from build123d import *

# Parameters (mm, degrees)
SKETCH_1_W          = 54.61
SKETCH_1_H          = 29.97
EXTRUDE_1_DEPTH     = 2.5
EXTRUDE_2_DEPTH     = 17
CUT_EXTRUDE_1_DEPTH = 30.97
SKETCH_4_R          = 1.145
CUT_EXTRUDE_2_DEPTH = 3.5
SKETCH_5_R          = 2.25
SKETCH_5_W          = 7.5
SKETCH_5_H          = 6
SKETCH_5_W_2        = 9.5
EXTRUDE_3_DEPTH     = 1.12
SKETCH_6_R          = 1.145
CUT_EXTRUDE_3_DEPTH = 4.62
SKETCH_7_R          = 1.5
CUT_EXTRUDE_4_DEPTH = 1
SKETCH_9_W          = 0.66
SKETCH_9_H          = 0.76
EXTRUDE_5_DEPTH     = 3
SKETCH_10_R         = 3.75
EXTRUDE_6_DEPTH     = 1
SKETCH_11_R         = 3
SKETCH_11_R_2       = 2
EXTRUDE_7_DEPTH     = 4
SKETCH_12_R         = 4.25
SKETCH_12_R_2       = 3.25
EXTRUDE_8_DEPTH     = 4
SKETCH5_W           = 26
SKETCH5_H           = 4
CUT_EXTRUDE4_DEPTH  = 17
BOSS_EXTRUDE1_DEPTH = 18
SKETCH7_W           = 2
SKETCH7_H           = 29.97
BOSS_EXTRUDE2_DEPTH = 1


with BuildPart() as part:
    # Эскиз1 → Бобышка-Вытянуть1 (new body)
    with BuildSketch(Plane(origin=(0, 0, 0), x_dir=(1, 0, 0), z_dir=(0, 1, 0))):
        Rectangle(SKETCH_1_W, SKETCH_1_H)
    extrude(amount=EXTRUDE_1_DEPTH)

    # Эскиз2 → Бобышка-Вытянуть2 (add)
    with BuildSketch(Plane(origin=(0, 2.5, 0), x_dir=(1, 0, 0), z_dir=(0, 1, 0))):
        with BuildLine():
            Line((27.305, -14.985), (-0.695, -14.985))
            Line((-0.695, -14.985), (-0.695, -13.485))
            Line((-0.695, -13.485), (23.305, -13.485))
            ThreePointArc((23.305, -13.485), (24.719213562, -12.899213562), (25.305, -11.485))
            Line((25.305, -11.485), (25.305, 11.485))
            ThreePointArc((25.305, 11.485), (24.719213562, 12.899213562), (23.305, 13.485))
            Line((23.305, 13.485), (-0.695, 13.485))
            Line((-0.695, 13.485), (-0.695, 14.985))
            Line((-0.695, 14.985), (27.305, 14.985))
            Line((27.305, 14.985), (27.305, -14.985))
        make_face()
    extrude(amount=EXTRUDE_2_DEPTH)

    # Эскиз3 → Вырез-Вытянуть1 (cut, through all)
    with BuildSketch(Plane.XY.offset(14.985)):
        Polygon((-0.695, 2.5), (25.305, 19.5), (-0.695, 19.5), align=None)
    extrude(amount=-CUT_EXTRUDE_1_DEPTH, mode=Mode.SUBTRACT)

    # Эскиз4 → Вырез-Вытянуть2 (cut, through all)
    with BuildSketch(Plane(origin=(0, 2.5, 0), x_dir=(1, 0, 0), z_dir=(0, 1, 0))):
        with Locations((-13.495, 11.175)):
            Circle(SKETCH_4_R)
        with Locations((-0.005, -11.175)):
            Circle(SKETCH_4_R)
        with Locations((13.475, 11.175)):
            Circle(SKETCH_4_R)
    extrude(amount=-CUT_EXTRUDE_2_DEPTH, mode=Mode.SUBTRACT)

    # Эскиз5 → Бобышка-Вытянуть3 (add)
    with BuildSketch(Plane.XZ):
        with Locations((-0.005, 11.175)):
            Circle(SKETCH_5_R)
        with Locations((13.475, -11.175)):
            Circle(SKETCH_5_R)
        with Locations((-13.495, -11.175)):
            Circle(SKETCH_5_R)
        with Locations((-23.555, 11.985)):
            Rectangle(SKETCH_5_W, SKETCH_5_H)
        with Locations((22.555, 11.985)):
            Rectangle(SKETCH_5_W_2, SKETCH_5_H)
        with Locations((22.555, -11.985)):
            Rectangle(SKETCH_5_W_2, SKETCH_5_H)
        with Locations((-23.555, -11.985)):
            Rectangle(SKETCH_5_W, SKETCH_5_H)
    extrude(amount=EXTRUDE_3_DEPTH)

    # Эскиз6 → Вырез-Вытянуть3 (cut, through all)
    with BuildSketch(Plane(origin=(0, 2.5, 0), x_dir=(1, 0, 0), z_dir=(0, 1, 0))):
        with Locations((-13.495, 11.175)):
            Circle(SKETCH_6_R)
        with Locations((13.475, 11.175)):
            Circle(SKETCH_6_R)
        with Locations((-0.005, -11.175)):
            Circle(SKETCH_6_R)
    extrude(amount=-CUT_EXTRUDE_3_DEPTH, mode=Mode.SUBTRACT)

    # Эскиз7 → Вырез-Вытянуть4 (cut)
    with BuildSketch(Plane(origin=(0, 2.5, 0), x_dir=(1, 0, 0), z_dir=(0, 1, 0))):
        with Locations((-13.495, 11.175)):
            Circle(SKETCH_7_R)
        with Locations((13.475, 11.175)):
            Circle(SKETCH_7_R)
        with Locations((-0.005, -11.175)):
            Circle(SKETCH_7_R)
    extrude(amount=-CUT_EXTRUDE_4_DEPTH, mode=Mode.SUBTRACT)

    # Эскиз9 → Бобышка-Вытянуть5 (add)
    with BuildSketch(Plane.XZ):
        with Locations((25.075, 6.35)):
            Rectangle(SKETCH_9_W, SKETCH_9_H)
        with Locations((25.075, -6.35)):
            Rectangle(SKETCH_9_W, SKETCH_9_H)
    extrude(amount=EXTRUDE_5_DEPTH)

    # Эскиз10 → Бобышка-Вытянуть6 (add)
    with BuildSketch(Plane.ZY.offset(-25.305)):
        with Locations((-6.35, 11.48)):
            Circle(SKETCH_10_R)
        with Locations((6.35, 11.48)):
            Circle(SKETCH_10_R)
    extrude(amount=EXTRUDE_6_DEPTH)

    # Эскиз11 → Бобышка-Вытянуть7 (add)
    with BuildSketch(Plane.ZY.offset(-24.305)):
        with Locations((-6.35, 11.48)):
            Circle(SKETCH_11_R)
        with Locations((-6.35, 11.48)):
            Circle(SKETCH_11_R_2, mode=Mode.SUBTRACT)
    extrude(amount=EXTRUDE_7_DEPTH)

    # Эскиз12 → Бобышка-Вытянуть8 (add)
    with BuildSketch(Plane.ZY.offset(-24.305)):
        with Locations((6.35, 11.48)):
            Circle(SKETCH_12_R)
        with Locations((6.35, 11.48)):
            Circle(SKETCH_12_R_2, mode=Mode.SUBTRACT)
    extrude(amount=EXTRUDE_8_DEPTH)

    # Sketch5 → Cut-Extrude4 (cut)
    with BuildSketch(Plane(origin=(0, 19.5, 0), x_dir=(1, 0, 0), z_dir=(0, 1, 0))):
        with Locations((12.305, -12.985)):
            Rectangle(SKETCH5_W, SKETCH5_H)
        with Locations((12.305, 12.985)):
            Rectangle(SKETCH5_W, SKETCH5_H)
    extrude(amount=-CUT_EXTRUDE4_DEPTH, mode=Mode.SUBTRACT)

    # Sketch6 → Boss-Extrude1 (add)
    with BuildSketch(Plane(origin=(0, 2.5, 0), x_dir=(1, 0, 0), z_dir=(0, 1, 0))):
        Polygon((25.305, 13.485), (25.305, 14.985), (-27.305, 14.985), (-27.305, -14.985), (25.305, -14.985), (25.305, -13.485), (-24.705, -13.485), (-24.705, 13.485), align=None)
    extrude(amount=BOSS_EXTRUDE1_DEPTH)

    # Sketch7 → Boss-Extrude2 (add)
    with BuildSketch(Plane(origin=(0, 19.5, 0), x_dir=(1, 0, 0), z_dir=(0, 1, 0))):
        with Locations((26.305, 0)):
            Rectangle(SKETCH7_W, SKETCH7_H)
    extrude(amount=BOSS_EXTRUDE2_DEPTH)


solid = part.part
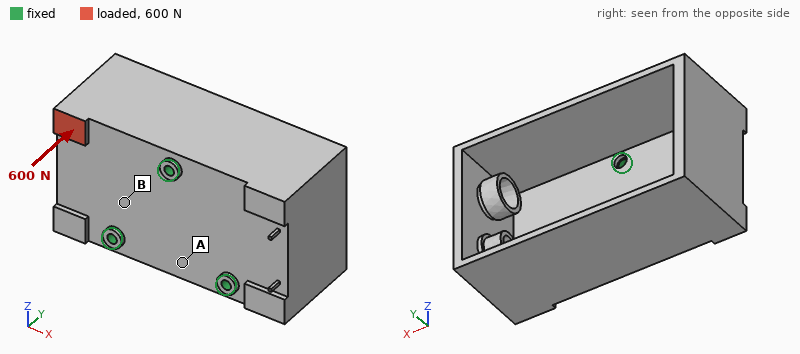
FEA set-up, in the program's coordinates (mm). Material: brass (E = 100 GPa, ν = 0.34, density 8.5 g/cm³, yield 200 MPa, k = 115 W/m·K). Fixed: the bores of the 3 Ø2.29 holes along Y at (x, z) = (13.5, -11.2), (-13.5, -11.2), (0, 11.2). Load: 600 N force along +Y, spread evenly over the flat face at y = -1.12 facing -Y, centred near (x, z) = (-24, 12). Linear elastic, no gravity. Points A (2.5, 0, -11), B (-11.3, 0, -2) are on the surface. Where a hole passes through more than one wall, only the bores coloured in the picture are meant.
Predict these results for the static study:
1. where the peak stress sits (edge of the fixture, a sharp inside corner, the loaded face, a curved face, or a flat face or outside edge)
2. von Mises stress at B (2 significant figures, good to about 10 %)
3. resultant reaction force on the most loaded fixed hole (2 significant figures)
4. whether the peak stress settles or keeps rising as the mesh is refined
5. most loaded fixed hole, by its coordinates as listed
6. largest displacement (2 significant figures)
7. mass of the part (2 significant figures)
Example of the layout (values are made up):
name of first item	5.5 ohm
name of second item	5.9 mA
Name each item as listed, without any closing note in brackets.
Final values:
where the peak stress sits	edge of the fixture
von Mises stress at B	58 MPa
resultant reaction force on the most loaded fixed hole	630 N
whether the peak stress settles or keeps rising as the mesh is refined	keeps rising
most loaded fixed hole, by its coordinates as listed	(0, 11.2)
largest displacement	0.27 mm
mass of the part	83 g
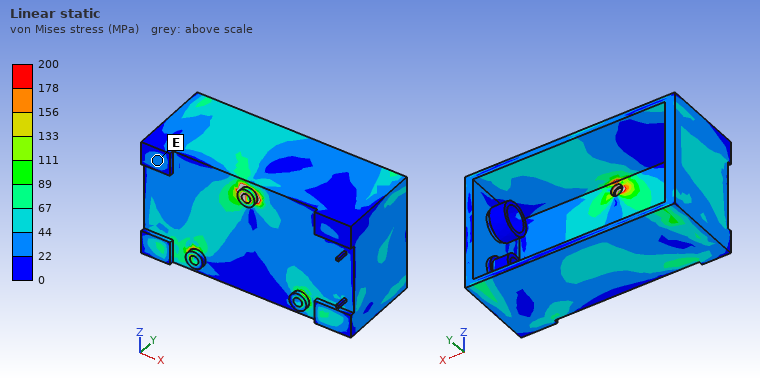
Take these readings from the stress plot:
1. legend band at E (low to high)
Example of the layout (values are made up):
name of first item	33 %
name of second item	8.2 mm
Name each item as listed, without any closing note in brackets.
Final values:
legend band at E	22 to 44 MPa
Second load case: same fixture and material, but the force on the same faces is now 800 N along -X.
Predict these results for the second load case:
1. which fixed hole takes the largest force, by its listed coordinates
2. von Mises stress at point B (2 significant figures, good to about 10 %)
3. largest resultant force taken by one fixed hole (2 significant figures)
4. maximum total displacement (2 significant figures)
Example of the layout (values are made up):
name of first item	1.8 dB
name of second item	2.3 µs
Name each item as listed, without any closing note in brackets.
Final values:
which fixed hole takes the largest force, by its listed coordinates	(0, 11.2)
von Mises stress at point B	12 MPa
largest resultant force taken by one fixed hole	700 N
maximum total displacement	36 µm
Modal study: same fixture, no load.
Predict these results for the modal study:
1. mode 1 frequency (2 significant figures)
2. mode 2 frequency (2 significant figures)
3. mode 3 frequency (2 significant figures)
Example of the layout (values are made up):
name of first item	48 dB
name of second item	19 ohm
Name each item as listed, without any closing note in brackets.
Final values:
mode 1 frequency	1700 Hz
mode 2 frequency	3400 Hz
mode 3 frequency	3500 Hz
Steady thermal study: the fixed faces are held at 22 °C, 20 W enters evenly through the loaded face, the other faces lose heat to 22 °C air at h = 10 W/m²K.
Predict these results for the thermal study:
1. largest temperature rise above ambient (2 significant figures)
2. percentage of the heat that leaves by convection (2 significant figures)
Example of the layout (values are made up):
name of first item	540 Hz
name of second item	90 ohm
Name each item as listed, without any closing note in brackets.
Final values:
largest temperature rise above ambient	58 K
percentage of the heat that leaves by convection	5.8 %
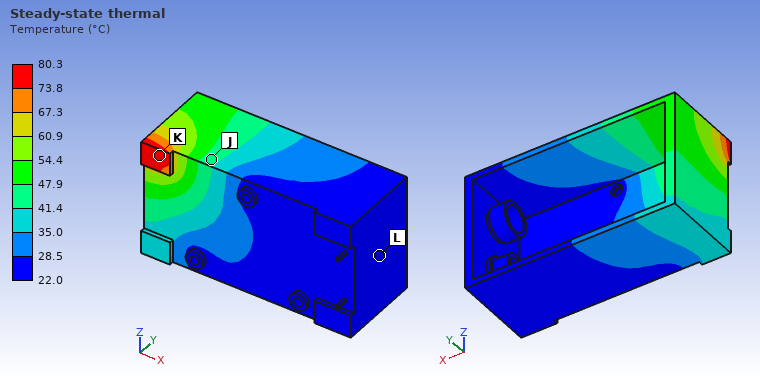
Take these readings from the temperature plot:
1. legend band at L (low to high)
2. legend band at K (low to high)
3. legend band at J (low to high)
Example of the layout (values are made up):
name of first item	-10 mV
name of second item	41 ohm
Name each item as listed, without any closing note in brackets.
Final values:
legend band at L	22.0 to 28.5 °C
legend band at K	73.8 to 80.3 °C
legend band at J	41.4 to 47.9 °C
